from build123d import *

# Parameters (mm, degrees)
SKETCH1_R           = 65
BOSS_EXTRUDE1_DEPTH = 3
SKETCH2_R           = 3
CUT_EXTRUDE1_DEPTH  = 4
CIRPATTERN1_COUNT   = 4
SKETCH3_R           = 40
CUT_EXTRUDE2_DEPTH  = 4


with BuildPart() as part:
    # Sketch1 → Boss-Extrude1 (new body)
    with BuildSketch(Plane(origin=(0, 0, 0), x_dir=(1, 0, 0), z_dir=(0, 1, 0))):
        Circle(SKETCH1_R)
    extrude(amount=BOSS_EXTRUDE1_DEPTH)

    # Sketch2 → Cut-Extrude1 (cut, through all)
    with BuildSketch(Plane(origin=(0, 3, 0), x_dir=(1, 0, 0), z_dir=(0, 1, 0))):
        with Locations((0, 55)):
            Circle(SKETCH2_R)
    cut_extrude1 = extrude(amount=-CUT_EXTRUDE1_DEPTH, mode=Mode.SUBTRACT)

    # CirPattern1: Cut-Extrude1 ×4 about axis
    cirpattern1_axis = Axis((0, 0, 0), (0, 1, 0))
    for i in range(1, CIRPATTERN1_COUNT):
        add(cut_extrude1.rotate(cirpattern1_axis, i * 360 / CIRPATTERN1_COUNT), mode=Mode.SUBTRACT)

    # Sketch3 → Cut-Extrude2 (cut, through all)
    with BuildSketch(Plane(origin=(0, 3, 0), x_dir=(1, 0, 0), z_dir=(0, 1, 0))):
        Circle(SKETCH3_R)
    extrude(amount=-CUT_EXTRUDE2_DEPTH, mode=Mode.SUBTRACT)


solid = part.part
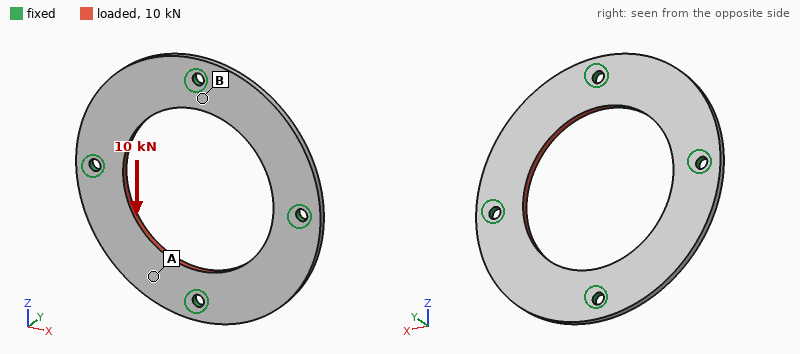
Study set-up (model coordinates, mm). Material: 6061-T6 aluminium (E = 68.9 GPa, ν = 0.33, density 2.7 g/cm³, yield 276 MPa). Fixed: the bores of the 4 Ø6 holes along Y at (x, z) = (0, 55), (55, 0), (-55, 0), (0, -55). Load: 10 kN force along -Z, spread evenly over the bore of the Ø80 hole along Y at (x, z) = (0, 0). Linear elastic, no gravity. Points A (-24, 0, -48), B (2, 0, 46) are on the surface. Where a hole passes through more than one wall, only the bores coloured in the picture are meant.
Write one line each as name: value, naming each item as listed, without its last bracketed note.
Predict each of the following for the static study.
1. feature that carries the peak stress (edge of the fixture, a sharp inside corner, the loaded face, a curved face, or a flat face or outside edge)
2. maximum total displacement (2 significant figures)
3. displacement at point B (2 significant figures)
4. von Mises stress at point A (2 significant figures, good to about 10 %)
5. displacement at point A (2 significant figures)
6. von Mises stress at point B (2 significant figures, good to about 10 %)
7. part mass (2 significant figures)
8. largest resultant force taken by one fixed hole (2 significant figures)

feature that carries the peak stress: edge of the fixture
maximum total displacement: 22 µm
displacement at point B: 3.6 µm
von Mises stress at point A: 16 MPa
displacement at point A: 16 µm
von Mises stress at point B: 37 MPa
part mass: 66 g
largest resultant force taken by one fixed hole: 3.0 kN
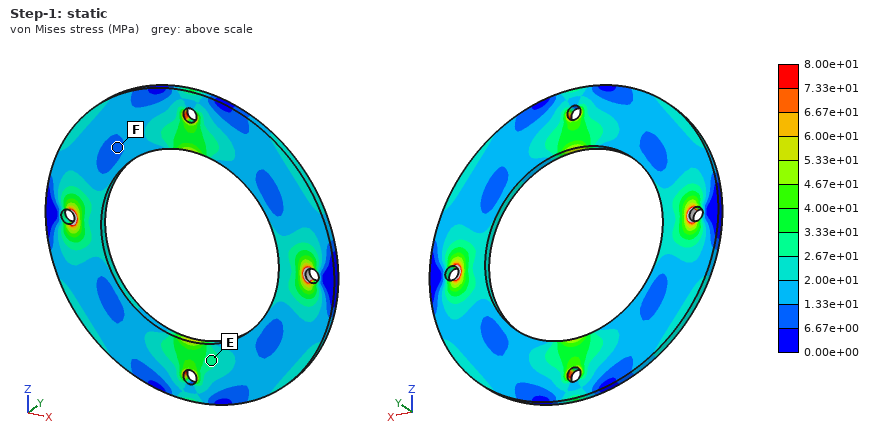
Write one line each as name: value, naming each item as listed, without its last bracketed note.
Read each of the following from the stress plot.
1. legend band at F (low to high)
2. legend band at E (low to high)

legend band at F: 6.67e+00 to 1.33e+01 MPa
legend band at E: 2.67e+01 to 3.33e+01 MPa
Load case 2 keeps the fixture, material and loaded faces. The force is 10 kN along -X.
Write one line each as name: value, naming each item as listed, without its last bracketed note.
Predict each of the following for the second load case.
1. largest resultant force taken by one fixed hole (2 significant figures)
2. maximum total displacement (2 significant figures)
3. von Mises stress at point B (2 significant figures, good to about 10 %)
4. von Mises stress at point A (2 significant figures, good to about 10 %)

largest resultant force taken by one fixed hole: 3.0 kN
maximum total displacement: 22 µm
von Mises stress at point B: 28 MPa
von Mises stress at point A: 17 MPa
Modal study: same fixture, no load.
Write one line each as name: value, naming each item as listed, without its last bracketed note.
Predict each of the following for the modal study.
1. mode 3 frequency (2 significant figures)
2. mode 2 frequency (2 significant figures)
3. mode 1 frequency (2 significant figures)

mode 3 frequency: 2100 Hz
mode 2 frequency: 2100 Hz
mode 1 frequency: 2100 Hz
